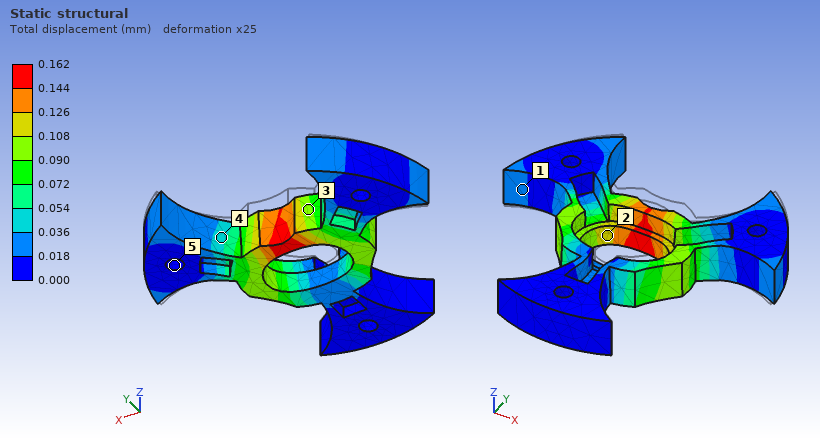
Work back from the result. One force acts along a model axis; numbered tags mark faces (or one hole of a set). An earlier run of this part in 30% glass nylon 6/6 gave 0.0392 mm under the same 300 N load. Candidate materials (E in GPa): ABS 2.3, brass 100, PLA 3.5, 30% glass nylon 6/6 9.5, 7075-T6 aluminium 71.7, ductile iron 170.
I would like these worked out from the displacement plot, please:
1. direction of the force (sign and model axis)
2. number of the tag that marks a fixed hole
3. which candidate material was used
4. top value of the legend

-Y
5
ABS
0.162 mm
